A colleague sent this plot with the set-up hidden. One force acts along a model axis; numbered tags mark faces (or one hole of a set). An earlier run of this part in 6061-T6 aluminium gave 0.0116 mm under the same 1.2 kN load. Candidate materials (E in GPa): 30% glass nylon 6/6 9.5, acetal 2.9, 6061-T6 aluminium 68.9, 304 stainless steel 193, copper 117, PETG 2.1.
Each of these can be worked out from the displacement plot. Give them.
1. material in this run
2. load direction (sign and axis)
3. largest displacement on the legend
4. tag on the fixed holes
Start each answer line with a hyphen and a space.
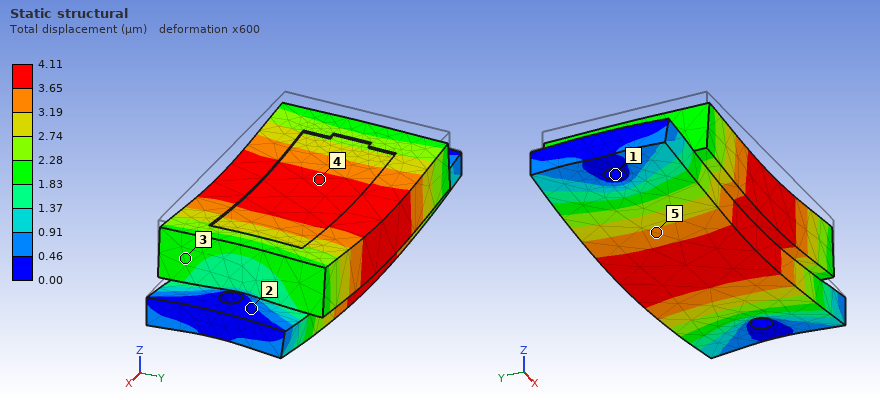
- 304 stainless steel
- -Z
- 4.11 µm
- 1
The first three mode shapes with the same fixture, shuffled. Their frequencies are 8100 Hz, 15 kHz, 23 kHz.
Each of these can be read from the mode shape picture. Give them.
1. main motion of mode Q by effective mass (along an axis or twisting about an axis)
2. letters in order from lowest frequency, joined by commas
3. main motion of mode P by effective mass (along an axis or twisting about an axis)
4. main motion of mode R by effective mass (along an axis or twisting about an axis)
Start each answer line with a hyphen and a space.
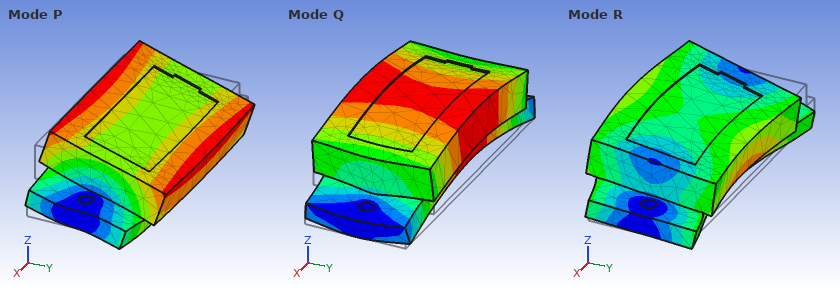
- along Z
- P, Q, R
- along Y
- along Y
